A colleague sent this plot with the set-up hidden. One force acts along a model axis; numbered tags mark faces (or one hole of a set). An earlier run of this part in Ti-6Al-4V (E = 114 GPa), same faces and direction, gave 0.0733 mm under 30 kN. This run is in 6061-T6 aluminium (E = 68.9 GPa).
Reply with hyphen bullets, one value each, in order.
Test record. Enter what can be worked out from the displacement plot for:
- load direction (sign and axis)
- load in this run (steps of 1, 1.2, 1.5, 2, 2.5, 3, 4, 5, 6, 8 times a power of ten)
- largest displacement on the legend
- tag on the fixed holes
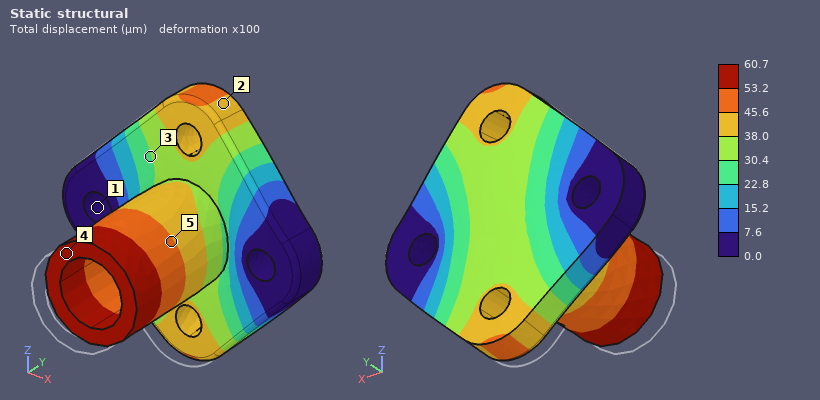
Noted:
- +Y
- 15 kN
- 60.7 µm
- 1
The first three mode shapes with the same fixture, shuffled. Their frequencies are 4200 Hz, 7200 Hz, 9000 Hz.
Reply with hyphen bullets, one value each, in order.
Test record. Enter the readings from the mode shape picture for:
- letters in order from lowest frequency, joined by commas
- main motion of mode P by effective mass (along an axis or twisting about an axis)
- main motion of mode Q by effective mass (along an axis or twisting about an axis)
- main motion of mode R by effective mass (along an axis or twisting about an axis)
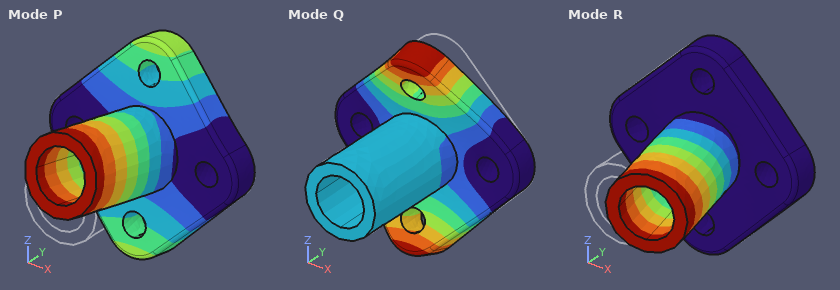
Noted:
- P, R, Q
- along Z
- along Y
- along X
